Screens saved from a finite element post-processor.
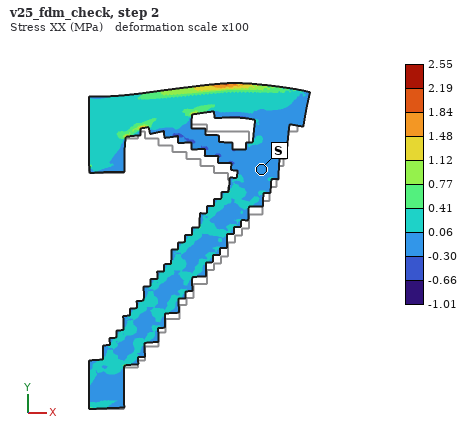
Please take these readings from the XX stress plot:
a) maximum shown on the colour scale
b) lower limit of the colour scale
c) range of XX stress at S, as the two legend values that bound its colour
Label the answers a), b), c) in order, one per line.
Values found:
a) 2.55 MPa
b) -1.01 MPa
c) -0.30 to 0.06 MPa
